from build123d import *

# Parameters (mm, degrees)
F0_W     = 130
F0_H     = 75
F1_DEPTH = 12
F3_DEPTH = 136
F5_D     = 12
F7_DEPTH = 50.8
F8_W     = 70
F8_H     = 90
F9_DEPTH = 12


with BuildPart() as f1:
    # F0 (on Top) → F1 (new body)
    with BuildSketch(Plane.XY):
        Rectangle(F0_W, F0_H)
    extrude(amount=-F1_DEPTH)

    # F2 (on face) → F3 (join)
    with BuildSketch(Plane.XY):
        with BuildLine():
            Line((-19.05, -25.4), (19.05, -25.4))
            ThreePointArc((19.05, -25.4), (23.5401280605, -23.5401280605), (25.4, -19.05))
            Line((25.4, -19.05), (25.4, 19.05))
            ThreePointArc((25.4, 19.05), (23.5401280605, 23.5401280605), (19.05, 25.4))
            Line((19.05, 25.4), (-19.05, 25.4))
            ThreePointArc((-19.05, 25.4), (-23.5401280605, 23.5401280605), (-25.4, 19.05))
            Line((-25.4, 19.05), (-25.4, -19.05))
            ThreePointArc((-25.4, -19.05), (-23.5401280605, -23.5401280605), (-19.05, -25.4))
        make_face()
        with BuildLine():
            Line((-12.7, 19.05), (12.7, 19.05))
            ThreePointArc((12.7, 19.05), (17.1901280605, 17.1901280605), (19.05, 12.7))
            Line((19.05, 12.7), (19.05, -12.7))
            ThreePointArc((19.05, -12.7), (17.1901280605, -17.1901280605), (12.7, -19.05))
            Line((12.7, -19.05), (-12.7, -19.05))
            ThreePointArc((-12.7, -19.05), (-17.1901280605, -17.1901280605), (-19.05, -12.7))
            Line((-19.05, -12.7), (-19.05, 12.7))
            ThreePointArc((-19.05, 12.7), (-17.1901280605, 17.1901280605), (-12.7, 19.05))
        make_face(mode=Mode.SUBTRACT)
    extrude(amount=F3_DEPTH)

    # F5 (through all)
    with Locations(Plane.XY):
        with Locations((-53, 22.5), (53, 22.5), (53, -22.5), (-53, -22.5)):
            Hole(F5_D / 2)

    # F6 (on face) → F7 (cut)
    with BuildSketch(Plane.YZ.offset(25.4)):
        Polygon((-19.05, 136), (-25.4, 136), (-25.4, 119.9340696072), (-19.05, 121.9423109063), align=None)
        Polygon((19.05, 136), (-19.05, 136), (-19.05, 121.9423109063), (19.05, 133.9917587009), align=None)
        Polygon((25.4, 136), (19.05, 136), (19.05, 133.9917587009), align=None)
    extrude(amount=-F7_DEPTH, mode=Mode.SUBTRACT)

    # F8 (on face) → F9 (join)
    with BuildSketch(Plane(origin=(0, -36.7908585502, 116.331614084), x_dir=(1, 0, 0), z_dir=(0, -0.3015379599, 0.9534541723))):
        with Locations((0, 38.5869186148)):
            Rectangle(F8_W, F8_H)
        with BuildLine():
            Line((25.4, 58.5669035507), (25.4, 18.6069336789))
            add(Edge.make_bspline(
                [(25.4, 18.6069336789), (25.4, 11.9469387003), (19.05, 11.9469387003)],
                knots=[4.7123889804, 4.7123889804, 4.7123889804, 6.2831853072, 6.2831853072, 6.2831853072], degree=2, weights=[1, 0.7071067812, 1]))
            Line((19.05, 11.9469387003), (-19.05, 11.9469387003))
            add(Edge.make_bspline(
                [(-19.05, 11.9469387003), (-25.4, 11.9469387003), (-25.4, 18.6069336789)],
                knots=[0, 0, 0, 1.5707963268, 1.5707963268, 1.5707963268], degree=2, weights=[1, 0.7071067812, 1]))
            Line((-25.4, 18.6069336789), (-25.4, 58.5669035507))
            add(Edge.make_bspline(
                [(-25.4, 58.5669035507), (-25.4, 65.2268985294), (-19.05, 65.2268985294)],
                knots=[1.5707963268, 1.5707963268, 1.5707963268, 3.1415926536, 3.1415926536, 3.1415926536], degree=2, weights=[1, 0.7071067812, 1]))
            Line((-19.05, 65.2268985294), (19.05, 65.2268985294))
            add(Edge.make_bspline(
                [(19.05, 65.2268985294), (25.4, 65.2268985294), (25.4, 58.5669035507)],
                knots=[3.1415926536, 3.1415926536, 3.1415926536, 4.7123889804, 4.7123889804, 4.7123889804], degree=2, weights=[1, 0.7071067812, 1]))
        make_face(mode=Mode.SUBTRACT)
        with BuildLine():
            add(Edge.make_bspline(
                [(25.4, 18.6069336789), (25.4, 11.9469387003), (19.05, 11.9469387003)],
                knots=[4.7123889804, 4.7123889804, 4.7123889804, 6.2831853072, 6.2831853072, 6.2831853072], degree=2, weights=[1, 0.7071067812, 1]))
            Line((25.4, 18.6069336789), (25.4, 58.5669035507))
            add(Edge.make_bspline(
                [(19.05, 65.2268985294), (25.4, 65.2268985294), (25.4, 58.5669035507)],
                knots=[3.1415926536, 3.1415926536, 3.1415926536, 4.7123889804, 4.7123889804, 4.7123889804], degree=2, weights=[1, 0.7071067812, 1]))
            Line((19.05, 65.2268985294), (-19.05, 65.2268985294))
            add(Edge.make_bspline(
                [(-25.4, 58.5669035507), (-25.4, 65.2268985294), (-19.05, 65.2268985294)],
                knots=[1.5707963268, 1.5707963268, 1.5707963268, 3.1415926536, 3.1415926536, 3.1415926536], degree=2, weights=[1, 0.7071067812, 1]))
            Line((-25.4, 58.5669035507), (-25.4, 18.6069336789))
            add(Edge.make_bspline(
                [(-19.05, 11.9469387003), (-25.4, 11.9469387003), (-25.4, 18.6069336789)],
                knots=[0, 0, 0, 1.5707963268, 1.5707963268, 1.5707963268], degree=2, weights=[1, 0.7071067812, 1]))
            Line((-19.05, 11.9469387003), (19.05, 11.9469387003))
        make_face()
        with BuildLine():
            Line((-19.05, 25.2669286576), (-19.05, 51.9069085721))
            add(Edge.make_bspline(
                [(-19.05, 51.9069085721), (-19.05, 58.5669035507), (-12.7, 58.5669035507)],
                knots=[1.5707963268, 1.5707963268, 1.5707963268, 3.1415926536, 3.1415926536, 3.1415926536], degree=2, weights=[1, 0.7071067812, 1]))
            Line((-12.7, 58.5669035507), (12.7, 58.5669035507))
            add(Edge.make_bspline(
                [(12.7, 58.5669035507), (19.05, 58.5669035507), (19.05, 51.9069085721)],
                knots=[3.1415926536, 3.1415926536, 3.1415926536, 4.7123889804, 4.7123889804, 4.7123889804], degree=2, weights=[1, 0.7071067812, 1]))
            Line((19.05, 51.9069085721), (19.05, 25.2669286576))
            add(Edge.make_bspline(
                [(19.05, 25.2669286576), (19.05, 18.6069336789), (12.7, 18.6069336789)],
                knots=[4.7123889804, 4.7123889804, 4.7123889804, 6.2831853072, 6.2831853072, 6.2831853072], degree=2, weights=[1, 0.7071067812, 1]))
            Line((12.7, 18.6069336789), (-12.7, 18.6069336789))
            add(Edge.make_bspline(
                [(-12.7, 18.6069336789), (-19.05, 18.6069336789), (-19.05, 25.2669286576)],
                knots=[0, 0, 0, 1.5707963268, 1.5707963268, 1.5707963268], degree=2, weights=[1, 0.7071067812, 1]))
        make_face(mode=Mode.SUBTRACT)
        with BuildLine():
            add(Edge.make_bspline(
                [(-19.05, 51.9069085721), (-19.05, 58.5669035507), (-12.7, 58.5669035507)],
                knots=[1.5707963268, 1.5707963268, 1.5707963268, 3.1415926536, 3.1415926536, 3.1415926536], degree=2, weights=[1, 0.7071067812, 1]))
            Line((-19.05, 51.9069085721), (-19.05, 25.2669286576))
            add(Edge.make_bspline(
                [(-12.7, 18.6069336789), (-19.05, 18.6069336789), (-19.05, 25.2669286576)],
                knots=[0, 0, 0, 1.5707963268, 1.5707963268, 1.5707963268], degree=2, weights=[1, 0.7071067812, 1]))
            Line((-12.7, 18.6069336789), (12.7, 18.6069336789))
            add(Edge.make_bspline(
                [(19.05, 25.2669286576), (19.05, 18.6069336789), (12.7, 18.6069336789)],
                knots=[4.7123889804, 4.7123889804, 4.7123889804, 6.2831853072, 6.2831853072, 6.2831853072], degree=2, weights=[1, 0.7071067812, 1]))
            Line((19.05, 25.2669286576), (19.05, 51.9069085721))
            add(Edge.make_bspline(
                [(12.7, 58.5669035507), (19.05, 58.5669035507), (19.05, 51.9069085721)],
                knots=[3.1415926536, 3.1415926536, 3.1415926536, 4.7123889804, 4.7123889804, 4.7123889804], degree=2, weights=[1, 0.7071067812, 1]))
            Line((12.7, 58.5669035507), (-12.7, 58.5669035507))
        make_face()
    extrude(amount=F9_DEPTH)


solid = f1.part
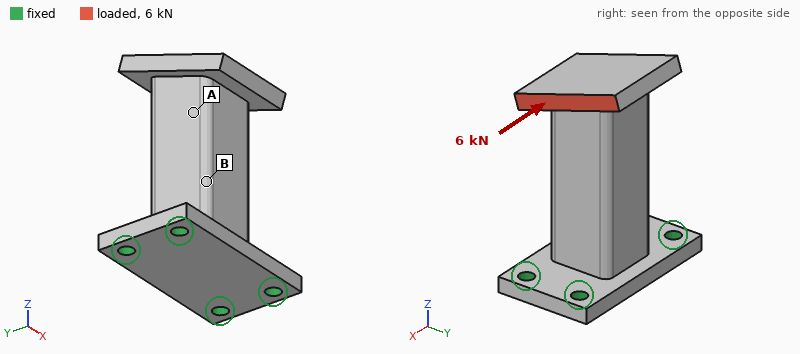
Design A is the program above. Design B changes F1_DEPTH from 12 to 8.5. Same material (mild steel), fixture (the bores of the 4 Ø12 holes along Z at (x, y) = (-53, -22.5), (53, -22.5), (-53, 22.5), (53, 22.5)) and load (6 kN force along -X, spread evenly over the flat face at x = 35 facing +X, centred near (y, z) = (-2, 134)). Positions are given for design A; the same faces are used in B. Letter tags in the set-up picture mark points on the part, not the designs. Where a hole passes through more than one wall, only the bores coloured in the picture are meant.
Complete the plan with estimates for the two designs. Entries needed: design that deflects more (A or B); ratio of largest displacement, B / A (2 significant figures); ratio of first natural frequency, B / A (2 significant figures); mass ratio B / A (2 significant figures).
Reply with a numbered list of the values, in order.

1. B
2. 1.5
3. 0.74
4. 0.90
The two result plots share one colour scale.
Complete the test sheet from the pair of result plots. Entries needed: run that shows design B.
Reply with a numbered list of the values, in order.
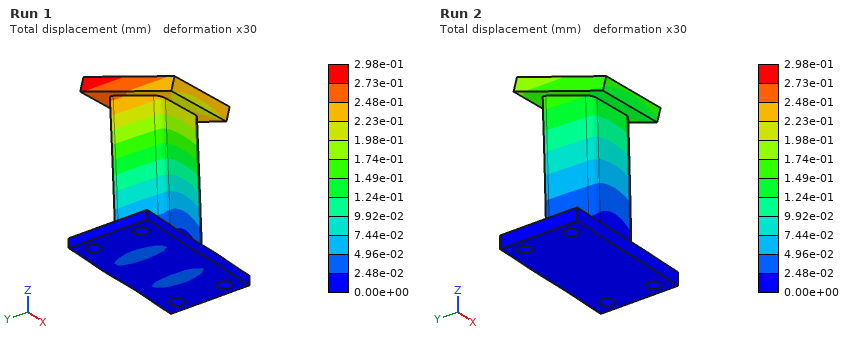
1. Run 1
